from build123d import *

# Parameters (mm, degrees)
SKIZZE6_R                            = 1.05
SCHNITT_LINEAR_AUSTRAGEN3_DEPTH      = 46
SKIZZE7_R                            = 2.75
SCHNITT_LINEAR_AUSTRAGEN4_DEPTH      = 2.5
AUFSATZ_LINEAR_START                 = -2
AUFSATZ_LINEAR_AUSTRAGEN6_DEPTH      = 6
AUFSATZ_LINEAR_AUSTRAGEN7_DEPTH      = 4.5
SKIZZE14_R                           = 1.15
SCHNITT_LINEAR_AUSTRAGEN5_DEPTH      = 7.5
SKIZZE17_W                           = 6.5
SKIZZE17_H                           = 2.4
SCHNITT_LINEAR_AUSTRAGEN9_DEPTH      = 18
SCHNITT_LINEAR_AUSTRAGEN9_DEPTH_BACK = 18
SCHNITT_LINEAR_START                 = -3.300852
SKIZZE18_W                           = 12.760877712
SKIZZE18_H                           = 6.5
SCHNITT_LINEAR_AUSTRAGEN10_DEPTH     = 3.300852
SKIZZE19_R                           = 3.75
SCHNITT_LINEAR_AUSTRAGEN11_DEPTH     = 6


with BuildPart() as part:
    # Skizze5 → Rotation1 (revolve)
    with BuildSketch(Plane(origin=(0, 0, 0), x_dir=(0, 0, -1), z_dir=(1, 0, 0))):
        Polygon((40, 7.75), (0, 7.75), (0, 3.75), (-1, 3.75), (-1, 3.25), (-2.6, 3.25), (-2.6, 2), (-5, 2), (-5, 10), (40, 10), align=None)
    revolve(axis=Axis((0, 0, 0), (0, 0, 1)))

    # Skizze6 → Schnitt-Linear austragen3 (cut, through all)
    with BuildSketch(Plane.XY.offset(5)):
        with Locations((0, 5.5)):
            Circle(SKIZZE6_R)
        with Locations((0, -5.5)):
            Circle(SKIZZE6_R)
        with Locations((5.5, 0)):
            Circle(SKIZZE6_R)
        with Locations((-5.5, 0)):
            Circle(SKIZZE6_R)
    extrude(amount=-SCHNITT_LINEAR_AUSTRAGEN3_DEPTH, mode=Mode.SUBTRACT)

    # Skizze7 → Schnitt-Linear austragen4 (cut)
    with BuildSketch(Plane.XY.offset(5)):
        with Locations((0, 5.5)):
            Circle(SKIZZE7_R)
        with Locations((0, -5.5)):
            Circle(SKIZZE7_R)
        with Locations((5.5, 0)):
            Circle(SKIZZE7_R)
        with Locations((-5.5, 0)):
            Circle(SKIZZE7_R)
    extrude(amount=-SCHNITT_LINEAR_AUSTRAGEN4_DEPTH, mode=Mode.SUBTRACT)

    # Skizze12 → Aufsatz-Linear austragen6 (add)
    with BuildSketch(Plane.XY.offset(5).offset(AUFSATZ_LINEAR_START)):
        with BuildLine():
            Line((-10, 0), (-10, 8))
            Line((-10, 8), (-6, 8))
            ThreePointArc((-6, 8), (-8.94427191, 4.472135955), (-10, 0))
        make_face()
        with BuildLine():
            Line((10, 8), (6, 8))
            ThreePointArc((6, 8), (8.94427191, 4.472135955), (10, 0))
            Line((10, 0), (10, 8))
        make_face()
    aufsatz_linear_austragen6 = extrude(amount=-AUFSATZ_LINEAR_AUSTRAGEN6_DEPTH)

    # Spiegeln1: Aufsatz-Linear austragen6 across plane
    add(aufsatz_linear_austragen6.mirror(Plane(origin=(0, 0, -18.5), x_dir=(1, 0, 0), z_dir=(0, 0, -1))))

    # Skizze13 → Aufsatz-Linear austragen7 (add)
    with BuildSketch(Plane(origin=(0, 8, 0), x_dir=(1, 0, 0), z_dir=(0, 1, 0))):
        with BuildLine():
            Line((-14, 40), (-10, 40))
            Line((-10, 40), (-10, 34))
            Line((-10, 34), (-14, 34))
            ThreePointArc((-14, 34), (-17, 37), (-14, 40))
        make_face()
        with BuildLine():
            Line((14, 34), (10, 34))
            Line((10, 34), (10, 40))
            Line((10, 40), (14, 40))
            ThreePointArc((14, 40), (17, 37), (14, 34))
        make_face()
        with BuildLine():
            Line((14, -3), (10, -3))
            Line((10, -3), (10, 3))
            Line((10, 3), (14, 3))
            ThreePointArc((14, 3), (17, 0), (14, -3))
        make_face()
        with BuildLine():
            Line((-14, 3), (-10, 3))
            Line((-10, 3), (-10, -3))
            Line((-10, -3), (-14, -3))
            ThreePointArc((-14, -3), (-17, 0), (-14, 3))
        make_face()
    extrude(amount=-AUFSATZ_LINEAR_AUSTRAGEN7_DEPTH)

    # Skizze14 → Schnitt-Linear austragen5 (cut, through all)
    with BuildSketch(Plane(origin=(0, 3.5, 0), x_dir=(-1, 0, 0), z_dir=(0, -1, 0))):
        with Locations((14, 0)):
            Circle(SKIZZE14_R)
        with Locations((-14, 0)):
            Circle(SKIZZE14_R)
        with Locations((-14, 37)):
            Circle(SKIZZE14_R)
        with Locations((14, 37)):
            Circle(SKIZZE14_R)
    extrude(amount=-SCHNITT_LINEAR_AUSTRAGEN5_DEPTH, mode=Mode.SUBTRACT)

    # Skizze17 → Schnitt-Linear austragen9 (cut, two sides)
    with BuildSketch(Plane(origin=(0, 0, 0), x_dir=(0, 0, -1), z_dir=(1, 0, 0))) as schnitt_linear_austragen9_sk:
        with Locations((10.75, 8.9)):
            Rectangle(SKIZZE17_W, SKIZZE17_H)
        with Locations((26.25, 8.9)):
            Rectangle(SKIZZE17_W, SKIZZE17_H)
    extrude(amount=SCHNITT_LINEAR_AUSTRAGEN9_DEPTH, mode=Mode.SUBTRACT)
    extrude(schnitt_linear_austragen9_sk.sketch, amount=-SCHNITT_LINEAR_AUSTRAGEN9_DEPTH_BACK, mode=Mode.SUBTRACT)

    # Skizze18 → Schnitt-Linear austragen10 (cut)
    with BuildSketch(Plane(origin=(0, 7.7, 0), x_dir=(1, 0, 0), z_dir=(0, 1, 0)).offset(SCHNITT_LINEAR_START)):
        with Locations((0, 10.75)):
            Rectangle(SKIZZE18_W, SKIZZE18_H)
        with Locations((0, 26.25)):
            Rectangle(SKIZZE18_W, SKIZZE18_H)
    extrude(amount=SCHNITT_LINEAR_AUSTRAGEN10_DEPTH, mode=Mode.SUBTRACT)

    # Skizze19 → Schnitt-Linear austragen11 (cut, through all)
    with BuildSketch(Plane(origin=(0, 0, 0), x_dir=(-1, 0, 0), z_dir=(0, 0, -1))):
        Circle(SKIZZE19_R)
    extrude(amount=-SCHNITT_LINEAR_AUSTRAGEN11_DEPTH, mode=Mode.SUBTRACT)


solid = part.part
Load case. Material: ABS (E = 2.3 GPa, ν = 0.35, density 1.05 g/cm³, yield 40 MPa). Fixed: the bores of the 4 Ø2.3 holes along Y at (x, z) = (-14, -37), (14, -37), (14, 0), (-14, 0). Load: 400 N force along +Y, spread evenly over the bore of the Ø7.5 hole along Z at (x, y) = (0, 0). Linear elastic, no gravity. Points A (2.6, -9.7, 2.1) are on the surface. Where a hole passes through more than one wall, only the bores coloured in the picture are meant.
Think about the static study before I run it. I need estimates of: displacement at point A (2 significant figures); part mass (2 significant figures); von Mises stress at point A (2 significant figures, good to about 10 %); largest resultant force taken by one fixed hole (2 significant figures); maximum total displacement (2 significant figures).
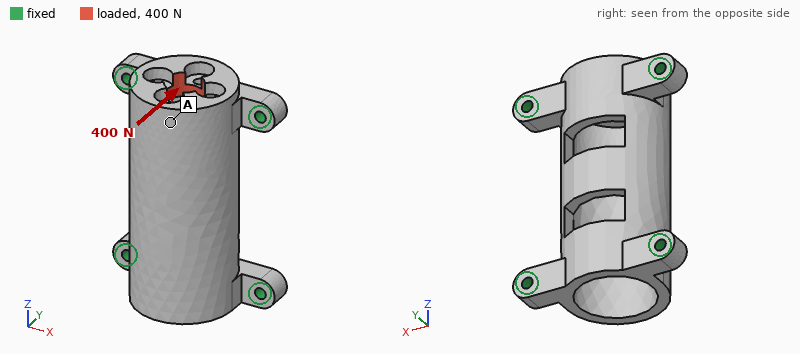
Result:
0.14 mm
6.9 g
4.0 MPa
210 N
0.19 mm
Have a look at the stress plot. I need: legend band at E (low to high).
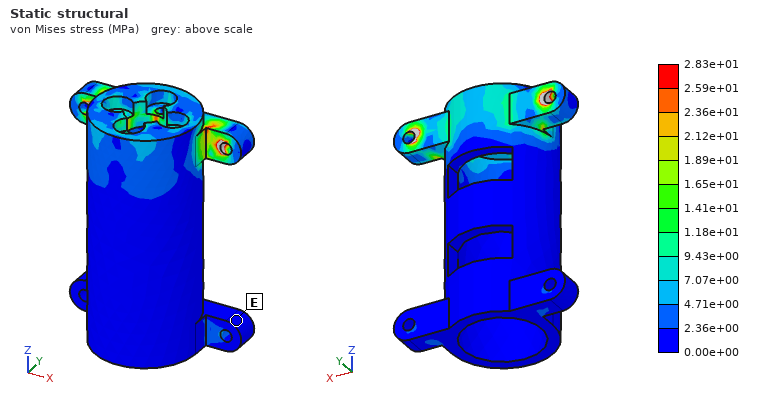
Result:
0.00e+00 to 2.36e+00 MPa
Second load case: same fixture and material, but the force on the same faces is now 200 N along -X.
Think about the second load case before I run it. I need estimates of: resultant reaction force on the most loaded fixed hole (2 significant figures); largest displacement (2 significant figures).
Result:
100 N
78 µm
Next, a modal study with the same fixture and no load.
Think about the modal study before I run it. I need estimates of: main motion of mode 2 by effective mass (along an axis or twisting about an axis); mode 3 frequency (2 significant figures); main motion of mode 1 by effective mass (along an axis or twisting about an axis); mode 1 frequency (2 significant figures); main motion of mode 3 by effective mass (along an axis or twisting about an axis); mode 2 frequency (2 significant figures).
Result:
along Z
4700 Hz
along X
3400 Hz
along Y
4300 Hz
